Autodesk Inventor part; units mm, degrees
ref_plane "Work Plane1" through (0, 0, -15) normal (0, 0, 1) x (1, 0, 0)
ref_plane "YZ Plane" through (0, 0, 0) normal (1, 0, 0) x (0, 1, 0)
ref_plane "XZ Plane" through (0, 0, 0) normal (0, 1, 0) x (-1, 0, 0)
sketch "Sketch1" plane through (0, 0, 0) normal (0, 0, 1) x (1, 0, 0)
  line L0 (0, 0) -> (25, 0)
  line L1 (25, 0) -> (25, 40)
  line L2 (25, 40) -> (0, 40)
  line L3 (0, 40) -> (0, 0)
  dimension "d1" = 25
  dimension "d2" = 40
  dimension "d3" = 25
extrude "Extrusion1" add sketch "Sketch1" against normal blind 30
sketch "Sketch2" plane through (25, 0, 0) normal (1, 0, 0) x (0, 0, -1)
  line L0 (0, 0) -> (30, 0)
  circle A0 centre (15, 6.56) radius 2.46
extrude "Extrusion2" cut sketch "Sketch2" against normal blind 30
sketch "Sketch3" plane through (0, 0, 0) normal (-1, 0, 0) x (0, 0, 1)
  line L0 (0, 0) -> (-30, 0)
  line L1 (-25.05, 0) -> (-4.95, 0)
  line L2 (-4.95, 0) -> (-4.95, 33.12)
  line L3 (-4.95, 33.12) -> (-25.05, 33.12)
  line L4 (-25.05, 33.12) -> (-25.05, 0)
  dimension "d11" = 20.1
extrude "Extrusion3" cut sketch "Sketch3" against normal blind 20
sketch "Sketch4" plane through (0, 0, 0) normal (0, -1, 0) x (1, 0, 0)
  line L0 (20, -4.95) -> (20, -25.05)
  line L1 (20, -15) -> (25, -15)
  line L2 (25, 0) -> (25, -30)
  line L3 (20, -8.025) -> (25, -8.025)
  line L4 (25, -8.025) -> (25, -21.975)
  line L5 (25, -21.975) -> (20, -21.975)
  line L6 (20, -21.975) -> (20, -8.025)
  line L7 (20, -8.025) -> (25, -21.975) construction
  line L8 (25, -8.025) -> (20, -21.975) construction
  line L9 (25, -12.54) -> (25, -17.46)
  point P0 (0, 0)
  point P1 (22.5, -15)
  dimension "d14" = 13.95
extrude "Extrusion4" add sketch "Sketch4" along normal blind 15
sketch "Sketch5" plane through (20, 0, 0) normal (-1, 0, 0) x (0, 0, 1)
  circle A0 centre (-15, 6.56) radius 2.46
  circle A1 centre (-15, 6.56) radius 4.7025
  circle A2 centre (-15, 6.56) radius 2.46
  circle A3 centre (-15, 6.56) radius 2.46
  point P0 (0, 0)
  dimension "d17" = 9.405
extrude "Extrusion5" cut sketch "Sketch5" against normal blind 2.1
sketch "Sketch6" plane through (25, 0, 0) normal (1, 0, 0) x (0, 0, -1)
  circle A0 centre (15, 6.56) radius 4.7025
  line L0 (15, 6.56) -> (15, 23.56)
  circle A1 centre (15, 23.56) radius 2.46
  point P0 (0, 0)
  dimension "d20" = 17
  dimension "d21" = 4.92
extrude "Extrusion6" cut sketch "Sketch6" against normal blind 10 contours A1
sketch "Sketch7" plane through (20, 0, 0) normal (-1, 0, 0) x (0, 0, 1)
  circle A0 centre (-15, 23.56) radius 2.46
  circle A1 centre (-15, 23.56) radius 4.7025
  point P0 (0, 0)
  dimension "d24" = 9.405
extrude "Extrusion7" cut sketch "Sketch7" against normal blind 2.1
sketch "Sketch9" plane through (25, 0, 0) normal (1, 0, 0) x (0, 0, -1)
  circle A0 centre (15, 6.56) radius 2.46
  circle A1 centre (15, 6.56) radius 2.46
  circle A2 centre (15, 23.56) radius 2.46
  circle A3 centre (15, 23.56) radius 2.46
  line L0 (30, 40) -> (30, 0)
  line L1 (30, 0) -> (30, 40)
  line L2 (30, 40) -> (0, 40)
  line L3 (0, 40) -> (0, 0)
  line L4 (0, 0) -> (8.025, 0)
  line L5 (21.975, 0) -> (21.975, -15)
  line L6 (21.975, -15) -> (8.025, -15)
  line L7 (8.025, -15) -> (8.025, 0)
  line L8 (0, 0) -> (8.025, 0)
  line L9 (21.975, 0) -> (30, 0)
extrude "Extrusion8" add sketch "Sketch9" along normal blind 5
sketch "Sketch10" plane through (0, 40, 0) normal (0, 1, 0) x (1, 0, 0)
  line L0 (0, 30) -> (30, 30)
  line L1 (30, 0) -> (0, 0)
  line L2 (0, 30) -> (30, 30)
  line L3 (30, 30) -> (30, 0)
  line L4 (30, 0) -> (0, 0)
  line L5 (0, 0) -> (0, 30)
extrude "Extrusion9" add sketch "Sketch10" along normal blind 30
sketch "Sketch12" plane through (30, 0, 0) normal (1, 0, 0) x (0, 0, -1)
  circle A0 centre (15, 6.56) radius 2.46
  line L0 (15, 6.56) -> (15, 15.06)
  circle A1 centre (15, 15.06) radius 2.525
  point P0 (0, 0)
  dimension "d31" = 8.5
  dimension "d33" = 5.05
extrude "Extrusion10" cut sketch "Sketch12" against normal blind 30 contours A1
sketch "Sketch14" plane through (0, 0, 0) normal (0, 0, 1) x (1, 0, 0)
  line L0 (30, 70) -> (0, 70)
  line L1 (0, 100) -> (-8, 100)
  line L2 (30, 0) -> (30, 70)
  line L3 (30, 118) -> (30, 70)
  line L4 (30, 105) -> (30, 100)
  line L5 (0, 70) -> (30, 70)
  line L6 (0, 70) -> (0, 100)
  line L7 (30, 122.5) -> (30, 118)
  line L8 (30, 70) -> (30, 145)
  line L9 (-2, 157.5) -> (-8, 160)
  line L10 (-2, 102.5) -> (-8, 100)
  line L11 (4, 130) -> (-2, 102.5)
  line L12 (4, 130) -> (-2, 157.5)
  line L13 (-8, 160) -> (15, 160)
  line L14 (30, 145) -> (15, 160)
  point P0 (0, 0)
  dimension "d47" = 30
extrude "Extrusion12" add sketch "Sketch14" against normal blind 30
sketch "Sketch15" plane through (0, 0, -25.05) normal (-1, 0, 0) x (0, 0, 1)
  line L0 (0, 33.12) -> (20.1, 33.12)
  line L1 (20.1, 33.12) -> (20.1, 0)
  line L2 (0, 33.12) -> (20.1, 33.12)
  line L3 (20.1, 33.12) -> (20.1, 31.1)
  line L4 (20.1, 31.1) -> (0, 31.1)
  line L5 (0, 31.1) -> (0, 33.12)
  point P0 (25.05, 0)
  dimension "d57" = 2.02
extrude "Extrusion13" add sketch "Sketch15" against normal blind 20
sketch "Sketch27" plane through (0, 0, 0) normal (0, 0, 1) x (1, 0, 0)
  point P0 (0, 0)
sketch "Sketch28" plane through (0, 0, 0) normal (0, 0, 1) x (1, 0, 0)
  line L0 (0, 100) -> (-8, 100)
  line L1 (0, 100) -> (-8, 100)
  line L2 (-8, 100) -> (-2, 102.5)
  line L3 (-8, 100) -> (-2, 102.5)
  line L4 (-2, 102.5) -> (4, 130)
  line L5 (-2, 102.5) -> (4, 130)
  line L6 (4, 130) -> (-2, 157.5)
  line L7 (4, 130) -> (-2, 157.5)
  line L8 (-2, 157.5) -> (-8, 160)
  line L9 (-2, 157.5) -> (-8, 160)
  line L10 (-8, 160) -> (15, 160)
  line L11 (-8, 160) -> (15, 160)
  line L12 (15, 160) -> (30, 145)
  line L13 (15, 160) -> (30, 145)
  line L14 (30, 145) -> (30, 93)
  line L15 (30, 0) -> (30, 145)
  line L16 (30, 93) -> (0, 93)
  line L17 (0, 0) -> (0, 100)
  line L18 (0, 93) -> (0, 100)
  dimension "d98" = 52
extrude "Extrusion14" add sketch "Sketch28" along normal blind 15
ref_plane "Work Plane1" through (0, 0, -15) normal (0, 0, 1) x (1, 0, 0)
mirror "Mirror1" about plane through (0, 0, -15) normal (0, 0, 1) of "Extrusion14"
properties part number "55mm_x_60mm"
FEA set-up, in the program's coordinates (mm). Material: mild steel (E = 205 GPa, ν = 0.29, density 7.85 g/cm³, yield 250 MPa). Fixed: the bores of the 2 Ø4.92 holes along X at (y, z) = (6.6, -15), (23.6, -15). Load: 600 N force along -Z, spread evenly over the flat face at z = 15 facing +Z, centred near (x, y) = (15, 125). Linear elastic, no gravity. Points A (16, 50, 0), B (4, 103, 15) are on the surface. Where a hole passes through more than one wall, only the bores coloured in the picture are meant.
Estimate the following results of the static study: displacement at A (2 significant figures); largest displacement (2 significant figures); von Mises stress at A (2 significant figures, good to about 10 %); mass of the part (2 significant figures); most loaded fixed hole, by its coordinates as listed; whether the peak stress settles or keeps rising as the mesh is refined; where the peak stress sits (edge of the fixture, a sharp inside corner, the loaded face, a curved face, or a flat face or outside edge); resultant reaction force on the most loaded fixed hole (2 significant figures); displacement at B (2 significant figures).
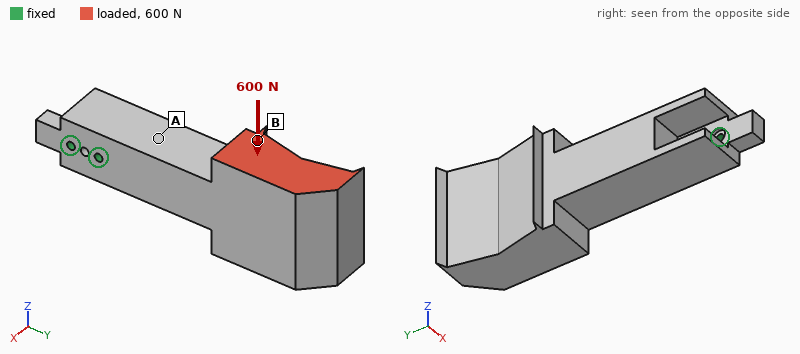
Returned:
11 µm
63 µm
10 MPa
1.4 kg
(23.6, -15)
keeps rising
edge of the fixture
3.2 kN
36 µm
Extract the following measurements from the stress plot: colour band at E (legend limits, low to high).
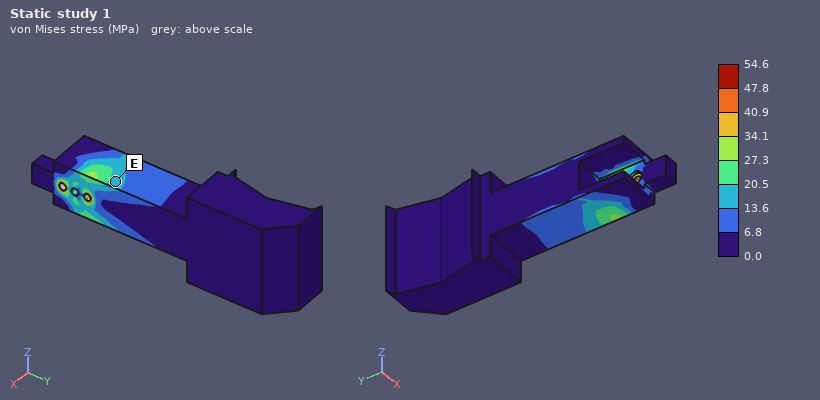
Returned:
13.6 to 20.5 MPa
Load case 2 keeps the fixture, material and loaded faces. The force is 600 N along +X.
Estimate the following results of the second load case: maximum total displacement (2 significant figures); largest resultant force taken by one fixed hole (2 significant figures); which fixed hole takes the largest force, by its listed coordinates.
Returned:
96 µm
3.0 kN
(23.6, -15)
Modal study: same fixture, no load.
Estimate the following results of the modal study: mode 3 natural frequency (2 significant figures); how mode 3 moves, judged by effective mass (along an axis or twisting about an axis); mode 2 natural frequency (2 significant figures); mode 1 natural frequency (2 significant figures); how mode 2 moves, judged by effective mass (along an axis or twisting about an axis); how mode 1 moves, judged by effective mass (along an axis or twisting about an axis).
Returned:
1700 Hz
twisting about Y
590 Hz
510 Hz
along Z
along X
